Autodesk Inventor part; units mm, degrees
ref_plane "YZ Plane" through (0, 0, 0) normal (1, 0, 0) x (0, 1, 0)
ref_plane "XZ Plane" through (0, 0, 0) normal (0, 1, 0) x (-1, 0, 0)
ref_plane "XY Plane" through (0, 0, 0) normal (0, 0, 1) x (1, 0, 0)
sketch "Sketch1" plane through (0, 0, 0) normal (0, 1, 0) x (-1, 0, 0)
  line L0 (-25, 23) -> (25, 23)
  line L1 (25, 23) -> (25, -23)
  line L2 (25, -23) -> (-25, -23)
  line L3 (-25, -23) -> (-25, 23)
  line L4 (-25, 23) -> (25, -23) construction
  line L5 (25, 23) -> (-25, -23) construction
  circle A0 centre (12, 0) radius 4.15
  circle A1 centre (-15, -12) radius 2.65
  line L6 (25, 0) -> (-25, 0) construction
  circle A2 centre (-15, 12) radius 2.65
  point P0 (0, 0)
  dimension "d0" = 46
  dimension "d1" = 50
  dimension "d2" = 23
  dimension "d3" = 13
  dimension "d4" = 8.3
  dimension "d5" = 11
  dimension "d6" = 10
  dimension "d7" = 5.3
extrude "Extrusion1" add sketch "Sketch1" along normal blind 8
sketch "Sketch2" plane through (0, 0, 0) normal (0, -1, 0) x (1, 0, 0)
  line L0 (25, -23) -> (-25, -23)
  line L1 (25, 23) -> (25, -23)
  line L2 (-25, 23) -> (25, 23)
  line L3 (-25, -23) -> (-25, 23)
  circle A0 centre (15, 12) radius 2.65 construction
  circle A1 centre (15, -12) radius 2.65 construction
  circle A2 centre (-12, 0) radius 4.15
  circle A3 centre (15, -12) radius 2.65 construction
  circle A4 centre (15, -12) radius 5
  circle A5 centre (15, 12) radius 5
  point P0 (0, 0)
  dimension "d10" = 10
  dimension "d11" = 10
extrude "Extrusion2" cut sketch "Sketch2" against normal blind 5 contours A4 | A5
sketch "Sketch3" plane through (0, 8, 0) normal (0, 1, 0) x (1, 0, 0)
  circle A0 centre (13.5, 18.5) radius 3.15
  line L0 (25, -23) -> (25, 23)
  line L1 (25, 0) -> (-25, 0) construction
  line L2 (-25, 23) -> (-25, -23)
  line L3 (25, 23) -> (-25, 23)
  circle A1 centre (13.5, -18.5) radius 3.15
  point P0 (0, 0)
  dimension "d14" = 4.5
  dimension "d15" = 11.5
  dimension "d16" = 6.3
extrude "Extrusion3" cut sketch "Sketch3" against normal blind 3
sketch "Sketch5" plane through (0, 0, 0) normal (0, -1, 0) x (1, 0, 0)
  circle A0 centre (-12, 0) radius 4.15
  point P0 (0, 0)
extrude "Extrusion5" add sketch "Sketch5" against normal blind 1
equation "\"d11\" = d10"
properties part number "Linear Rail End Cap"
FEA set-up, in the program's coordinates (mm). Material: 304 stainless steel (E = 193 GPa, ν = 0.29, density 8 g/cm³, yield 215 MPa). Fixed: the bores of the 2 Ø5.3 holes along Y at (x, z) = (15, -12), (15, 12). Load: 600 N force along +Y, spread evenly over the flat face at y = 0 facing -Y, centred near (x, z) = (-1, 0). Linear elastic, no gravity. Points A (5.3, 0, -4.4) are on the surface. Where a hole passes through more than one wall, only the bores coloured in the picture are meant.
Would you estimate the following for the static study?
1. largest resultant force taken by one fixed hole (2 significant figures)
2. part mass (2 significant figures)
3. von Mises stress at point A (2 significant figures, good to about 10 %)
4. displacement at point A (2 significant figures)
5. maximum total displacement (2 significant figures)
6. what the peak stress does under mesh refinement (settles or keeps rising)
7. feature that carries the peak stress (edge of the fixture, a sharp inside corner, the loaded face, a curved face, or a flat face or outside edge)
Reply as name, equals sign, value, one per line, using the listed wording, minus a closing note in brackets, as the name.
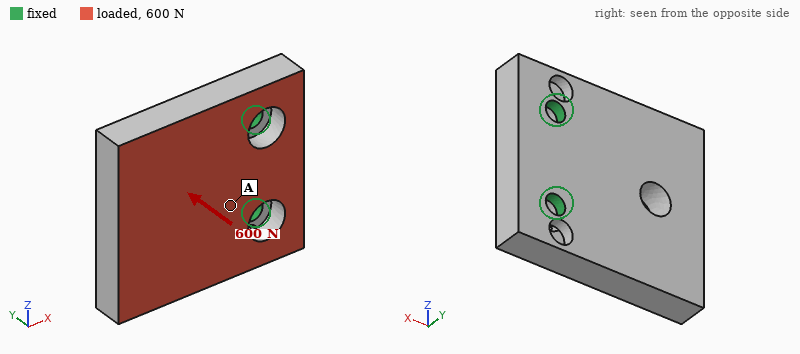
largest resultant force taken by one fixed hole = 300 N
part mass = 140 g
von Mises stress at point A = 16 MPa
displacement at point A = 8.2 µm
maximum total displacement = 35 µm
what the peak stress does under mesh refinement = keeps rising
feature that carries the peak stress = edge of the fixture
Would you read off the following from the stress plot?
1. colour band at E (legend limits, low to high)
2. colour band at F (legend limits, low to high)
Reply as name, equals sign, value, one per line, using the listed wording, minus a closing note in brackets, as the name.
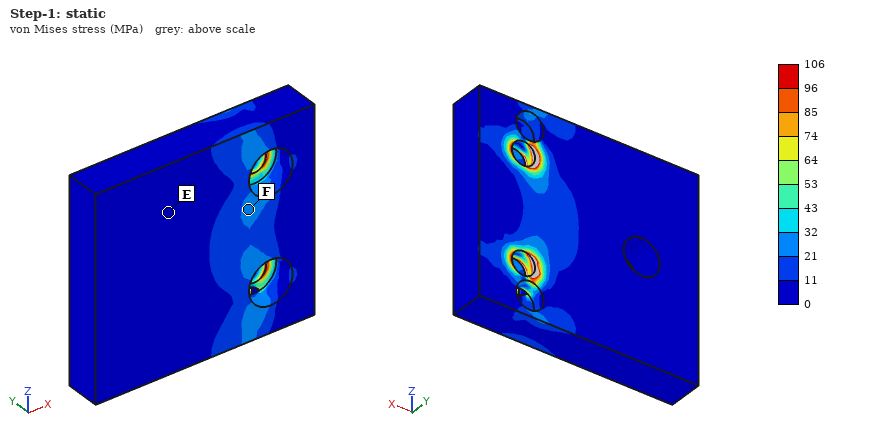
colour band at E = 0 to 11 MPa
colour band at F = 21 to 32 MPa
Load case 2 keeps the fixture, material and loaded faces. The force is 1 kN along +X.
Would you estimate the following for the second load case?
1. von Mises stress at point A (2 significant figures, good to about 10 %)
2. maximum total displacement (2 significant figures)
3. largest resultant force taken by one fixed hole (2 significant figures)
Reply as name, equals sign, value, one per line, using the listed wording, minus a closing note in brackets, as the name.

von Mises stress at point A = 9.9 MPa
maximum total displacement = 22 µm
largest resultant force taken by one fixed hole = 500 N
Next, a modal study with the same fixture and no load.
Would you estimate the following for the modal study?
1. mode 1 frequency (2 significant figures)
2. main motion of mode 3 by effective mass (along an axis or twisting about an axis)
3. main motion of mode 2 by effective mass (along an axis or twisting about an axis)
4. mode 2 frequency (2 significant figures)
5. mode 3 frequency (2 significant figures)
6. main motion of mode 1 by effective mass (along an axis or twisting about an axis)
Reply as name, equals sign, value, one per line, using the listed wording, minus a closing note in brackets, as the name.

mode 1 frequency = 2200 Hz
main motion of mode 3 by effective mass = along Z
main motion of mode 2 by effective mass = twisting about X
mode 2 frequency = 6100 Hz
mode 3 frequency = 8700 Hz
main motion of mode 1 by effective mass = along Y
